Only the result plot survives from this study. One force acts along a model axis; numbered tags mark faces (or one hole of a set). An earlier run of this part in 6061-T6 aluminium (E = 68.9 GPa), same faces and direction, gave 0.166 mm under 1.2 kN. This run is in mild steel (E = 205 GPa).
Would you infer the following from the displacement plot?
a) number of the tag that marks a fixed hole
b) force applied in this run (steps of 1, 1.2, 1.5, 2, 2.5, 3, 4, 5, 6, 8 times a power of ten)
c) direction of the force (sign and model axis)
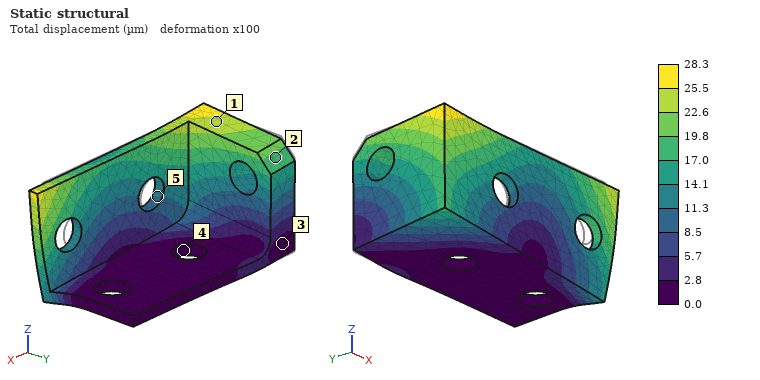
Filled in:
4
600 N
+X
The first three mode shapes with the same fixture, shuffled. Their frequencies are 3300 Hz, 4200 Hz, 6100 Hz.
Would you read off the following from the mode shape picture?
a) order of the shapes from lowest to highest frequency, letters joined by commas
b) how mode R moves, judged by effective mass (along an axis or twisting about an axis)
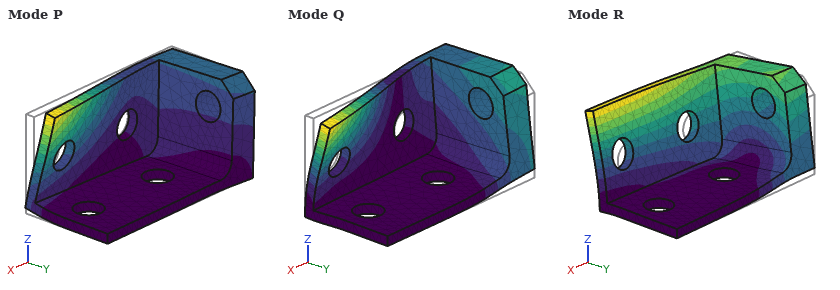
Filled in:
R, P, Q
along Y
